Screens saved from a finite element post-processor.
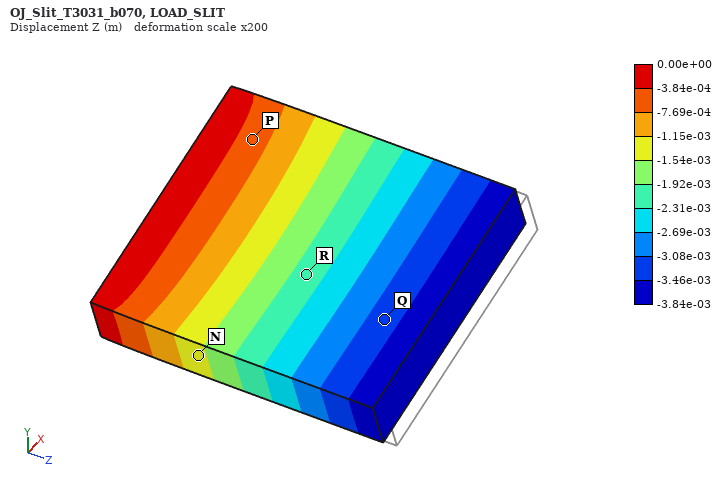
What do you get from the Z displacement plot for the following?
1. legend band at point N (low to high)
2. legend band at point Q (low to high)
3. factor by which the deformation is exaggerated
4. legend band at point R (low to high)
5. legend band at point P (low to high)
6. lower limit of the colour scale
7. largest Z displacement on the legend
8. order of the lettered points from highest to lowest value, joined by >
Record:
-1.54e-03 to -1.15e-03 m
-3.46e-03 to -3.08e-03 m
200
-2.31e-03 to -1.92e-03 m
-7.69e-04 to -3.84e-04 m
-3.84e-03 m
0.00e+00 m
P > N > R > Q
